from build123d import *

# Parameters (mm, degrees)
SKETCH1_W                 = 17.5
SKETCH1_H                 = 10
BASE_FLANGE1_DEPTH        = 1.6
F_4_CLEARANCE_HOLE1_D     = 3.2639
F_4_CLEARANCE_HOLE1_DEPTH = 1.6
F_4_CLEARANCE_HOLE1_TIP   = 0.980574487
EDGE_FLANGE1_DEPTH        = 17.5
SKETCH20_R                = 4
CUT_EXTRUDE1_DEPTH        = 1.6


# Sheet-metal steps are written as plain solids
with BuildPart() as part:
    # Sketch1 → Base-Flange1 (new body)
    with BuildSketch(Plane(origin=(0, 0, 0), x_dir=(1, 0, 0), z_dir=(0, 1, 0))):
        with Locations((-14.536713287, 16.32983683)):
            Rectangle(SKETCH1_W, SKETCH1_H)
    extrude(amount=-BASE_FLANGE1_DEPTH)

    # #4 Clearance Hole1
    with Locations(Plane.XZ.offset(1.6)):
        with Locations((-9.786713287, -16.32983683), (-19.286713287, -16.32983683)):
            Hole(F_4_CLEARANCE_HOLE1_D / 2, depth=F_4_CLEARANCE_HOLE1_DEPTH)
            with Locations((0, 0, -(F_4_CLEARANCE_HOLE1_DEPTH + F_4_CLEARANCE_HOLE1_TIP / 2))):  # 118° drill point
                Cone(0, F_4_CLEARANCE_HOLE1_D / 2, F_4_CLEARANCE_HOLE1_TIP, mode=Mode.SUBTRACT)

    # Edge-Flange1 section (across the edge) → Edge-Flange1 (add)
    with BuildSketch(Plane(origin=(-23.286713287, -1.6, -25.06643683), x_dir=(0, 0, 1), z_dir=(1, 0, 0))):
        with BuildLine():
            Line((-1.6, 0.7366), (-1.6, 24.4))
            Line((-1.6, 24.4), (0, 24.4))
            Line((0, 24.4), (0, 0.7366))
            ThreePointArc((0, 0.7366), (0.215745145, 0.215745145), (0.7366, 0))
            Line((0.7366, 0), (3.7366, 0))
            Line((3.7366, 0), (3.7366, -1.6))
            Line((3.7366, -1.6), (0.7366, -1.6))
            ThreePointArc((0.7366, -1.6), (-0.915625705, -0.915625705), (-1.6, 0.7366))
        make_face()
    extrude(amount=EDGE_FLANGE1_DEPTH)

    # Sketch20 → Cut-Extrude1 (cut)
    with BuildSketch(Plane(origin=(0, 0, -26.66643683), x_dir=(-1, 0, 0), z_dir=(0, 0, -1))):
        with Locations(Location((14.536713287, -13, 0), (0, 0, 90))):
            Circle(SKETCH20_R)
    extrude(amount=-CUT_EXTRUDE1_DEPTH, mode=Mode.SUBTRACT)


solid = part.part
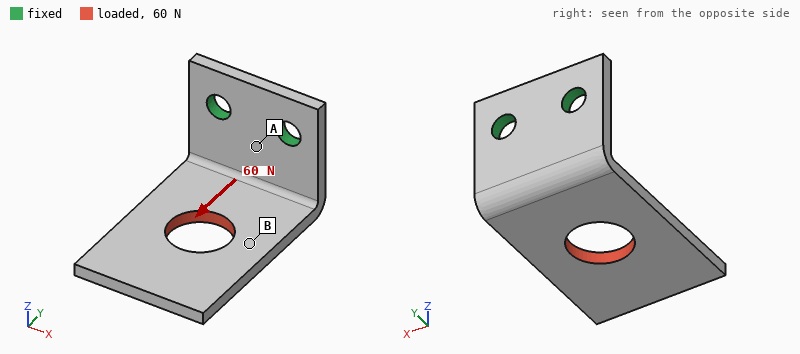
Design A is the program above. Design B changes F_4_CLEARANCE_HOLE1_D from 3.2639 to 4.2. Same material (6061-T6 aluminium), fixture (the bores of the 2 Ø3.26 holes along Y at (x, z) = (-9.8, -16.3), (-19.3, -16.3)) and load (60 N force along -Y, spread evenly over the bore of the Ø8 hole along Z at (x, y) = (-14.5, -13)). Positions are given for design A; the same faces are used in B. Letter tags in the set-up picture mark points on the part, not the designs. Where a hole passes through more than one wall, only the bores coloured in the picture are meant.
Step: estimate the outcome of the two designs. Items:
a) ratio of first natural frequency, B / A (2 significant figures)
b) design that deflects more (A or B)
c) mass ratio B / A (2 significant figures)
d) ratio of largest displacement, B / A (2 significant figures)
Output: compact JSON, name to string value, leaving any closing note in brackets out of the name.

{"ratio of first natural frequency, B / A": "1.0", "design that deflects more": "A", "mass ratio B / A": "0.98", "ratio of largest displacement, B / A": "0.87"}
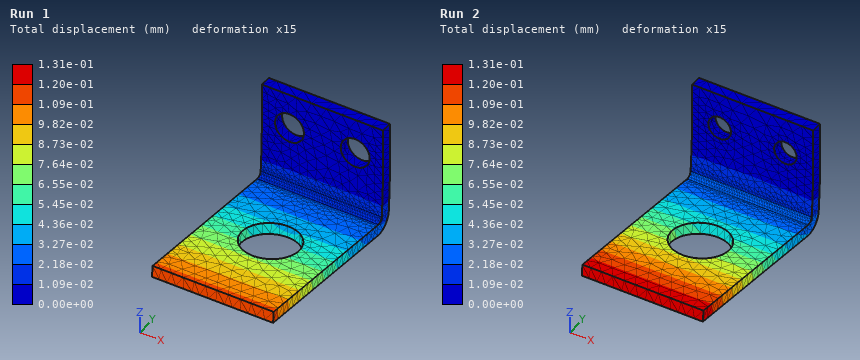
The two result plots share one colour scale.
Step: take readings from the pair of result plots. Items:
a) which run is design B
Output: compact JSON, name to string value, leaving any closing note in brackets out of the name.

{"which run is design B": "Run 1"}
